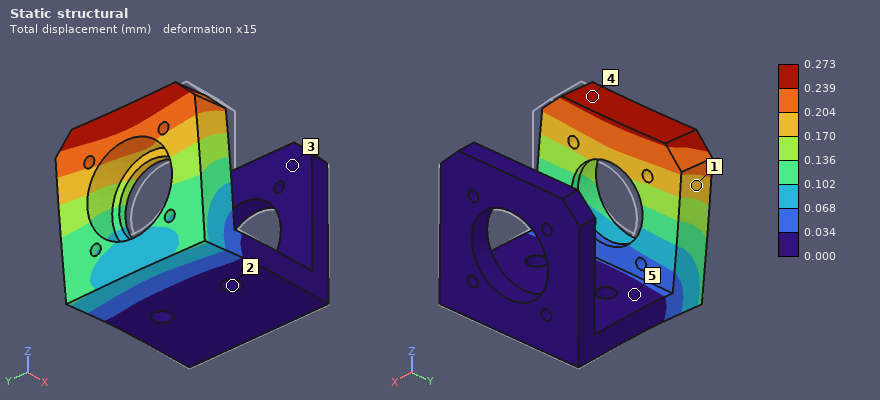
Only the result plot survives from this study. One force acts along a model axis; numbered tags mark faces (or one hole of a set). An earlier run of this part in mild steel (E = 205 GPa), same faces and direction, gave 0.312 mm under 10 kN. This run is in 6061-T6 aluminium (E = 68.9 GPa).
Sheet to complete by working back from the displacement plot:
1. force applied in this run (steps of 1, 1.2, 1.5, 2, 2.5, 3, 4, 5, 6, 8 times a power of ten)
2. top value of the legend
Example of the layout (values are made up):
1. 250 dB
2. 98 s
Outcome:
1. 3 kN
2. 0.273 mm
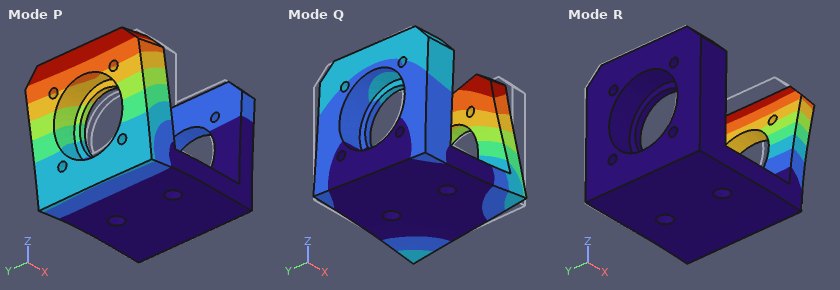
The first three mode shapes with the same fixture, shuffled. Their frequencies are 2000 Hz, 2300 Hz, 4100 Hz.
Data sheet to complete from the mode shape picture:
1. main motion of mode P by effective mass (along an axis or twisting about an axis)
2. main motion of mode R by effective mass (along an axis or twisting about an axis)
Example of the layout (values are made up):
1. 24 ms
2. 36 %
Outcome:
1. along X
2. along X
